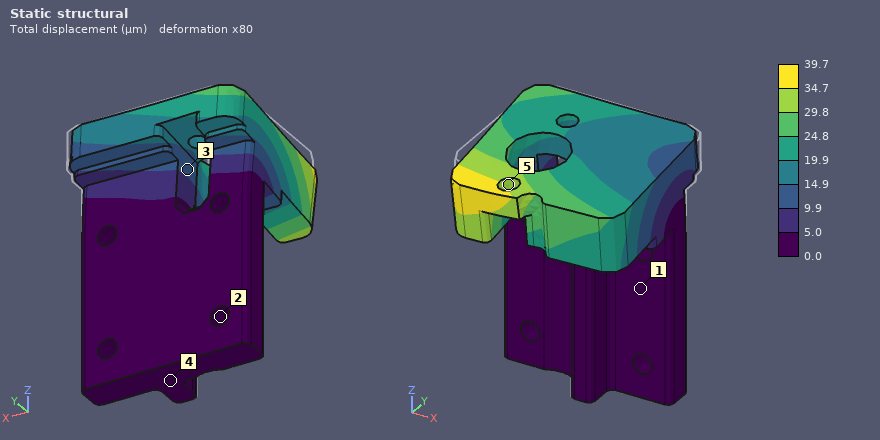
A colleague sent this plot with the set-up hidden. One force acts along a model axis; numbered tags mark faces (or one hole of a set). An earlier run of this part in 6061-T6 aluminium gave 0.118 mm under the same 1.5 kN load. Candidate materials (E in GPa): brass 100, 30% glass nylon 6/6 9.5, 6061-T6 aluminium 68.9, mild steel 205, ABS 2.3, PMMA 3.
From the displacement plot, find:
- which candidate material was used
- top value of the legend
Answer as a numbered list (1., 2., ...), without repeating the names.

1. mild steel
2. 39.7 µm
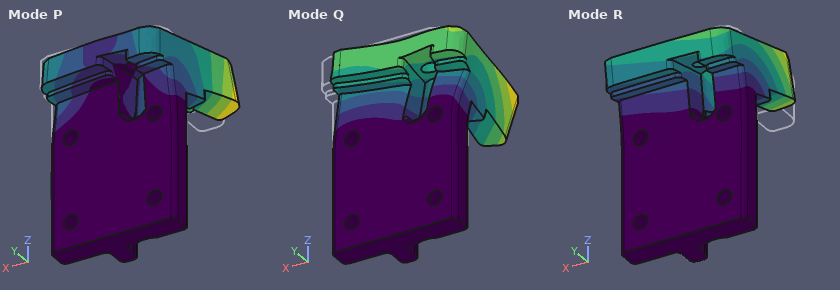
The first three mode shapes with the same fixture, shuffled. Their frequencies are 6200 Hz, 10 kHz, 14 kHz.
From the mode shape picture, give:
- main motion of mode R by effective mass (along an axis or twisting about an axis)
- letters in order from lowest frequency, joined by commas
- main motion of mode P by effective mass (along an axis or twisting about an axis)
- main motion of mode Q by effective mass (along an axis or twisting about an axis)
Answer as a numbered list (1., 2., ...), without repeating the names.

1. along Y
2. R, P, Q
3. along X
4. along X
